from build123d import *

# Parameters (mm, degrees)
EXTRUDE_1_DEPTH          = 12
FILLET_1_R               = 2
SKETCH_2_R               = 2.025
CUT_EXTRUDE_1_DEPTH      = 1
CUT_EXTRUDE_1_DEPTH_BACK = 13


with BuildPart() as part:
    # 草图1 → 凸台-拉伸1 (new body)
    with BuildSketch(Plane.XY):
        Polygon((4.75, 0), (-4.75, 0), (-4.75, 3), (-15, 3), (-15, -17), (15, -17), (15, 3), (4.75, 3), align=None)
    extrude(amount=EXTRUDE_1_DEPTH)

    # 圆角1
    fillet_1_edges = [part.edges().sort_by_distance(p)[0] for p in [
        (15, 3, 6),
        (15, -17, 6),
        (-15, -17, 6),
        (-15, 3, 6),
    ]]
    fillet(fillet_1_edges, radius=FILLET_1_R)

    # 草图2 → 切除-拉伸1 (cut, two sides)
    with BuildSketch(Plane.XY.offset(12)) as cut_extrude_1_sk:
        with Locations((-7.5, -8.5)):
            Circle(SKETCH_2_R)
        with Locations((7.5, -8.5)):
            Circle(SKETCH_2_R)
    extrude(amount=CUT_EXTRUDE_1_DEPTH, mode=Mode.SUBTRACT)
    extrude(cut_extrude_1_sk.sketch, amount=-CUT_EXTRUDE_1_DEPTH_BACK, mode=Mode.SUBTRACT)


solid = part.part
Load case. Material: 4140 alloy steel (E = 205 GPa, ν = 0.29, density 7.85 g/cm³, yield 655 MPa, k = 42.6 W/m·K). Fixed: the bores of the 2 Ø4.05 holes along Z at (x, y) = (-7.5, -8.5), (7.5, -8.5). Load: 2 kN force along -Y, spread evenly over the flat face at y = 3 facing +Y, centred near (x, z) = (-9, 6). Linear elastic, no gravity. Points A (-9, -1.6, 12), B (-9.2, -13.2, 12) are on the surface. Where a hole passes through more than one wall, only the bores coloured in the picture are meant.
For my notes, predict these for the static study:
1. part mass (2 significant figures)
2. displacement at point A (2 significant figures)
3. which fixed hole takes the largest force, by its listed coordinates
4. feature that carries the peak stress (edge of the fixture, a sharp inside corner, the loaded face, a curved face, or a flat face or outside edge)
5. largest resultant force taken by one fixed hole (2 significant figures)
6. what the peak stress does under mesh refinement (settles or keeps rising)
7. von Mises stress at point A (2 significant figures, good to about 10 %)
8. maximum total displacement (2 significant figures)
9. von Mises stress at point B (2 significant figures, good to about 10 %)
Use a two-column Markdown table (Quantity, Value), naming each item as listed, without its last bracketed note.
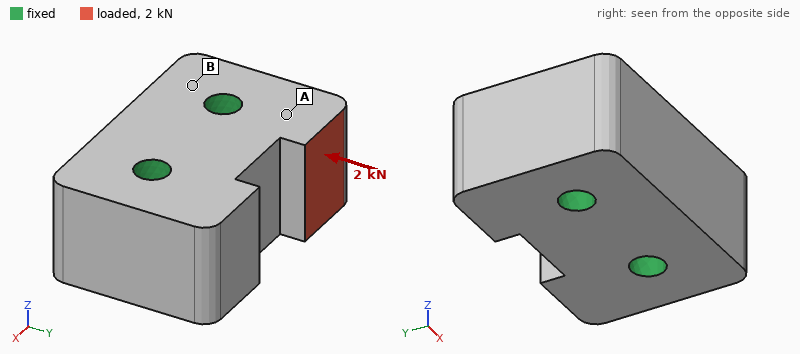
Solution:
| Quantity | Value |
|---|---|
| part mass | 51 g |
| displacement at point A | 0.70 µm |
| which fixed hole takes the largest force, by its listed coordinates | (-7.5, -8.5) |
| feature that carries the peak stress | edge of the fixture |
| largest resultant force taken by one fixed hole | 2.0 kN |
| what the peak stress does under mesh refinement | keeps rising |
| von Mises stress at point A | 22 MPa |
| maximum total displacement | 1.2 µm |
| von Mises stress at point B | 4.7 MPa |
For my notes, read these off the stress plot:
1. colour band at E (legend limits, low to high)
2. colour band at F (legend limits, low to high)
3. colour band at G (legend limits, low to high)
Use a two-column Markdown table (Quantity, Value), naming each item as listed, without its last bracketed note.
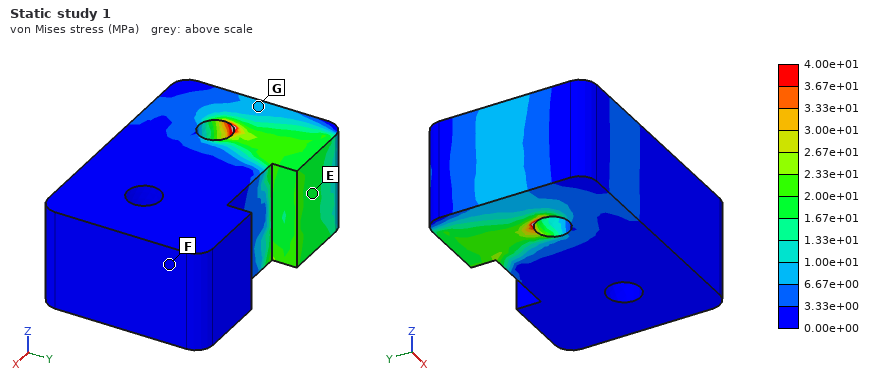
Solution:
| Quantity | Value |
|---|---|
| colour band at E | 1.67e+01 to 2.00e+01 MPa |
| colour band at F | 0.00e+00 to 3.33e+00 MPa |
| colour band at G | 6.67e+00 to 1.00e+01 MPa |
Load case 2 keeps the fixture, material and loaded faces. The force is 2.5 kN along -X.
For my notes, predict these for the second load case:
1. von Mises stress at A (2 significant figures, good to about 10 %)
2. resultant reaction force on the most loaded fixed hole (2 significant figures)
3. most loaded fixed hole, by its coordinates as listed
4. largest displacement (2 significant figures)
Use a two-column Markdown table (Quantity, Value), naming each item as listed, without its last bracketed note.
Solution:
| Quantity | Value |
|---|---|
| von Mises stress at A | 31 MPa |
| resultant reaction force on the most loaded fixed hole | 1.9 kN |
| most loaded fixed hole, by its coordinates as listed | (-7.5, -8.5) |
| largest displacement | 5.6 µm |
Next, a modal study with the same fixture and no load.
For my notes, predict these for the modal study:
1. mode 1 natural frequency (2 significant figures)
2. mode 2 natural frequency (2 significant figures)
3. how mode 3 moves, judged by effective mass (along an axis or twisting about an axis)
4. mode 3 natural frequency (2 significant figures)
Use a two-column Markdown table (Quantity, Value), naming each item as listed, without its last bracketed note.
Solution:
| Quantity | Value |
|---|---|
| mode 1 natural frequency | 50 kHz |
| mode 2 natural frequency | 50 kHz |
| how mode 3 moves, judged by effective mass | twisting about Y |
| mode 3 natural frequency | 53 kHz |
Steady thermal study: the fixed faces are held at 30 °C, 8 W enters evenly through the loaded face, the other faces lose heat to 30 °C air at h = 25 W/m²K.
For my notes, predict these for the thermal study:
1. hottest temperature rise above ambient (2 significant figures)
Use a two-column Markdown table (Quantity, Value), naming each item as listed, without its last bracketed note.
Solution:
| Quantity | Value |
|---|---|
| hottest temperature rise above ambient | 15 K |
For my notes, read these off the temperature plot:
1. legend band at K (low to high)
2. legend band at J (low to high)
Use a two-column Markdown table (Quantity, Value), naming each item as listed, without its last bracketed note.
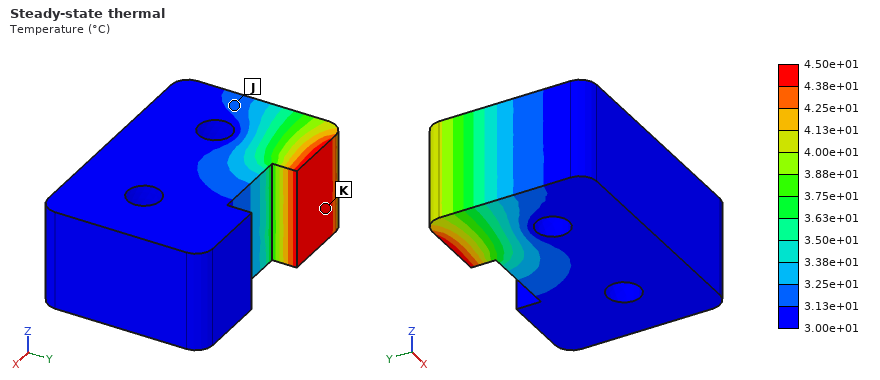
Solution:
| Quantity | Value |
|---|---|
| legend band at K | 4.38e+01 to 4.50e+01 °C |
| legend band at J | 3.13e+01 to 3.25e+01 °C |
